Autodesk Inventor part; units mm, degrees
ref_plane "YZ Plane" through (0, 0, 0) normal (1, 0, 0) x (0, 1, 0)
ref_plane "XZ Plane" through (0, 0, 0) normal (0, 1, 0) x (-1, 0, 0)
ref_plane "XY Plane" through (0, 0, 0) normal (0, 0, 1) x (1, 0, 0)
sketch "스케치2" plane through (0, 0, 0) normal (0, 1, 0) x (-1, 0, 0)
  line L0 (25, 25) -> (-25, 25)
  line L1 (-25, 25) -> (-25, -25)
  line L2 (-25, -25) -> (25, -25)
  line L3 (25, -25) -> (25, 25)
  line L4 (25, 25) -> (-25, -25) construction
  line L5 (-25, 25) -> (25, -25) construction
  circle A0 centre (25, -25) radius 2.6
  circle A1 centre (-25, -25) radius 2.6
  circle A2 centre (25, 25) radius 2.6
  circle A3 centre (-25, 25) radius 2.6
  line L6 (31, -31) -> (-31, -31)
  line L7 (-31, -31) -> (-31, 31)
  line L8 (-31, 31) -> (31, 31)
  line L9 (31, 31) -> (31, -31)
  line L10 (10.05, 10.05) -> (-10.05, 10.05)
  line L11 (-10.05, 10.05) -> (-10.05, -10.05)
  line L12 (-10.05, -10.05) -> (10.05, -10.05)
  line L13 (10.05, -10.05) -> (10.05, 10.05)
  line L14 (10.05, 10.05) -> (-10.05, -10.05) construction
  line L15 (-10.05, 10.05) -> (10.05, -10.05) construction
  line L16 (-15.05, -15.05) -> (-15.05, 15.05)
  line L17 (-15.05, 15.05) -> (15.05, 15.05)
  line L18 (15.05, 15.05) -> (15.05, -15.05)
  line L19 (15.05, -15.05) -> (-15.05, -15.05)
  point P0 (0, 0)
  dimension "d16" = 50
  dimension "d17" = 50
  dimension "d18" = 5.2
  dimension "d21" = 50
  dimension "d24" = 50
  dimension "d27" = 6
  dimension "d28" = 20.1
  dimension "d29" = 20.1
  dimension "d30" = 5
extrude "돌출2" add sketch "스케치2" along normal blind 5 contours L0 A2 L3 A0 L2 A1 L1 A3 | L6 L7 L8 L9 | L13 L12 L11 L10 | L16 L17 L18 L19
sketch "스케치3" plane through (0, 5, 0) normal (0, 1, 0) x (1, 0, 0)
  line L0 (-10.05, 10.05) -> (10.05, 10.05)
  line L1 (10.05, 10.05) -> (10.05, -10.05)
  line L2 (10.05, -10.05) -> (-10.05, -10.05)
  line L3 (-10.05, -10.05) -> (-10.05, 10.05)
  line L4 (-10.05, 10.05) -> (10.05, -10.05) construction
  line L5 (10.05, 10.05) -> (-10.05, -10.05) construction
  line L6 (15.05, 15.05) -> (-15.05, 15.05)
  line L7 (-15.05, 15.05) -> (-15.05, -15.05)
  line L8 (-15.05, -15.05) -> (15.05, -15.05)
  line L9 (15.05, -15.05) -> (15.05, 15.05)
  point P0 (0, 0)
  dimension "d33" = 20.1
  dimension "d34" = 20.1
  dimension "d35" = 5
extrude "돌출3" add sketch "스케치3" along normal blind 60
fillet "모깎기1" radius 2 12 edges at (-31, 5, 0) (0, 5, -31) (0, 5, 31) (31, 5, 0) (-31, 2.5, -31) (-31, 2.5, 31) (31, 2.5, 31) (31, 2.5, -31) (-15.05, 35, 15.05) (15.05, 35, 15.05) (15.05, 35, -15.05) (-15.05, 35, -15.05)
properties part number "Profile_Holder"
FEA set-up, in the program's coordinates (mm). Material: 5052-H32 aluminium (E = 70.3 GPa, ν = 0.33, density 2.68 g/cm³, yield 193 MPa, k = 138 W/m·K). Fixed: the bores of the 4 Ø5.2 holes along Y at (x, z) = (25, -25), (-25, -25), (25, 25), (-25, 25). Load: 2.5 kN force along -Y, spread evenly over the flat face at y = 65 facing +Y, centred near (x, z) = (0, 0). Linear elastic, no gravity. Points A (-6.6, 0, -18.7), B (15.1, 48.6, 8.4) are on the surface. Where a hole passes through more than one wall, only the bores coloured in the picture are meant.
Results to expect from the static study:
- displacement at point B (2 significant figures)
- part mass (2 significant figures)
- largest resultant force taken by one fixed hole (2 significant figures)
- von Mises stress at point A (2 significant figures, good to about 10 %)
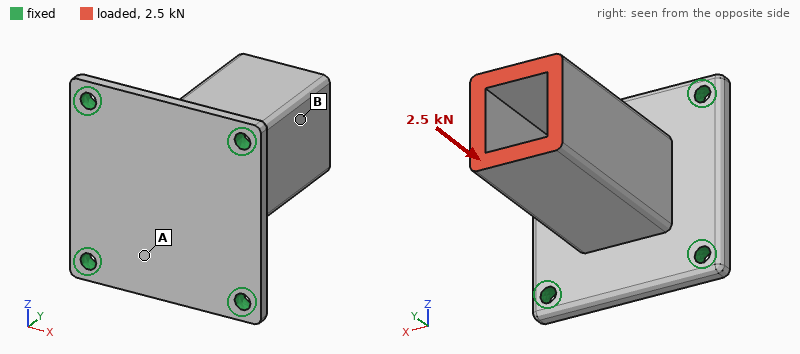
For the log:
30 µm
130 g
650 N
20 MPa
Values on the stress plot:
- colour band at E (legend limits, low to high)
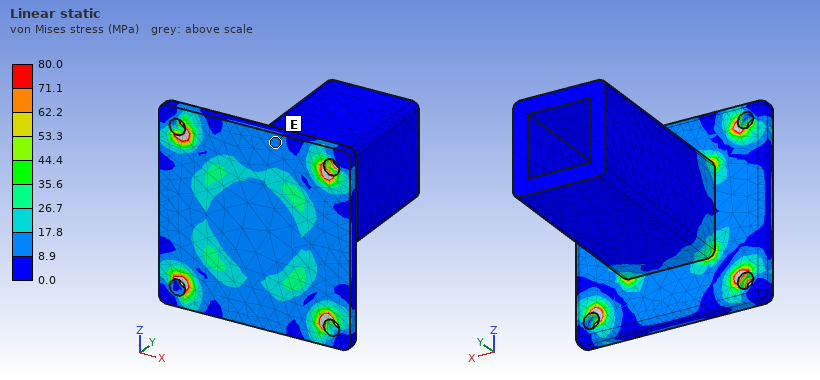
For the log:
8.9 to 17.8 MPa
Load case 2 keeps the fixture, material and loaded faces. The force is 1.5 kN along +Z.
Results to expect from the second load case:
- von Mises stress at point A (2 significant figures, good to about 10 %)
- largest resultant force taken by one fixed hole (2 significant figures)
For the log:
49 MPa
1.2 kN
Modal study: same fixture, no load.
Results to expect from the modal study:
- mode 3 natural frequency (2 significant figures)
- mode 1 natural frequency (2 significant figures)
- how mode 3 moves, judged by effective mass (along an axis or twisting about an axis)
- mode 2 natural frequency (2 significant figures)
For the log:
4600 Hz
2600 Hz
along Y
2600 Hz
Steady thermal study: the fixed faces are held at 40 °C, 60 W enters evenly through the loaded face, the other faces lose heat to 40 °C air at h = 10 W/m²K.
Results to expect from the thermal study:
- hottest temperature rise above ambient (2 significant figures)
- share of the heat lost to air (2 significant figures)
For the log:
67 K
9.6 %
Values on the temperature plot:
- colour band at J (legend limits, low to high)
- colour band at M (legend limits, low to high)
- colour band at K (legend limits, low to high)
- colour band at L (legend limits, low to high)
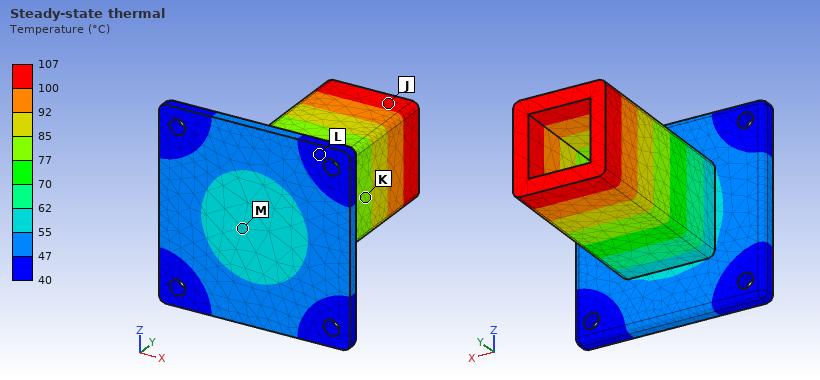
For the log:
100 to 107 °C
55 to 62 °C
77 to 85 °C
40 to 47 °C
